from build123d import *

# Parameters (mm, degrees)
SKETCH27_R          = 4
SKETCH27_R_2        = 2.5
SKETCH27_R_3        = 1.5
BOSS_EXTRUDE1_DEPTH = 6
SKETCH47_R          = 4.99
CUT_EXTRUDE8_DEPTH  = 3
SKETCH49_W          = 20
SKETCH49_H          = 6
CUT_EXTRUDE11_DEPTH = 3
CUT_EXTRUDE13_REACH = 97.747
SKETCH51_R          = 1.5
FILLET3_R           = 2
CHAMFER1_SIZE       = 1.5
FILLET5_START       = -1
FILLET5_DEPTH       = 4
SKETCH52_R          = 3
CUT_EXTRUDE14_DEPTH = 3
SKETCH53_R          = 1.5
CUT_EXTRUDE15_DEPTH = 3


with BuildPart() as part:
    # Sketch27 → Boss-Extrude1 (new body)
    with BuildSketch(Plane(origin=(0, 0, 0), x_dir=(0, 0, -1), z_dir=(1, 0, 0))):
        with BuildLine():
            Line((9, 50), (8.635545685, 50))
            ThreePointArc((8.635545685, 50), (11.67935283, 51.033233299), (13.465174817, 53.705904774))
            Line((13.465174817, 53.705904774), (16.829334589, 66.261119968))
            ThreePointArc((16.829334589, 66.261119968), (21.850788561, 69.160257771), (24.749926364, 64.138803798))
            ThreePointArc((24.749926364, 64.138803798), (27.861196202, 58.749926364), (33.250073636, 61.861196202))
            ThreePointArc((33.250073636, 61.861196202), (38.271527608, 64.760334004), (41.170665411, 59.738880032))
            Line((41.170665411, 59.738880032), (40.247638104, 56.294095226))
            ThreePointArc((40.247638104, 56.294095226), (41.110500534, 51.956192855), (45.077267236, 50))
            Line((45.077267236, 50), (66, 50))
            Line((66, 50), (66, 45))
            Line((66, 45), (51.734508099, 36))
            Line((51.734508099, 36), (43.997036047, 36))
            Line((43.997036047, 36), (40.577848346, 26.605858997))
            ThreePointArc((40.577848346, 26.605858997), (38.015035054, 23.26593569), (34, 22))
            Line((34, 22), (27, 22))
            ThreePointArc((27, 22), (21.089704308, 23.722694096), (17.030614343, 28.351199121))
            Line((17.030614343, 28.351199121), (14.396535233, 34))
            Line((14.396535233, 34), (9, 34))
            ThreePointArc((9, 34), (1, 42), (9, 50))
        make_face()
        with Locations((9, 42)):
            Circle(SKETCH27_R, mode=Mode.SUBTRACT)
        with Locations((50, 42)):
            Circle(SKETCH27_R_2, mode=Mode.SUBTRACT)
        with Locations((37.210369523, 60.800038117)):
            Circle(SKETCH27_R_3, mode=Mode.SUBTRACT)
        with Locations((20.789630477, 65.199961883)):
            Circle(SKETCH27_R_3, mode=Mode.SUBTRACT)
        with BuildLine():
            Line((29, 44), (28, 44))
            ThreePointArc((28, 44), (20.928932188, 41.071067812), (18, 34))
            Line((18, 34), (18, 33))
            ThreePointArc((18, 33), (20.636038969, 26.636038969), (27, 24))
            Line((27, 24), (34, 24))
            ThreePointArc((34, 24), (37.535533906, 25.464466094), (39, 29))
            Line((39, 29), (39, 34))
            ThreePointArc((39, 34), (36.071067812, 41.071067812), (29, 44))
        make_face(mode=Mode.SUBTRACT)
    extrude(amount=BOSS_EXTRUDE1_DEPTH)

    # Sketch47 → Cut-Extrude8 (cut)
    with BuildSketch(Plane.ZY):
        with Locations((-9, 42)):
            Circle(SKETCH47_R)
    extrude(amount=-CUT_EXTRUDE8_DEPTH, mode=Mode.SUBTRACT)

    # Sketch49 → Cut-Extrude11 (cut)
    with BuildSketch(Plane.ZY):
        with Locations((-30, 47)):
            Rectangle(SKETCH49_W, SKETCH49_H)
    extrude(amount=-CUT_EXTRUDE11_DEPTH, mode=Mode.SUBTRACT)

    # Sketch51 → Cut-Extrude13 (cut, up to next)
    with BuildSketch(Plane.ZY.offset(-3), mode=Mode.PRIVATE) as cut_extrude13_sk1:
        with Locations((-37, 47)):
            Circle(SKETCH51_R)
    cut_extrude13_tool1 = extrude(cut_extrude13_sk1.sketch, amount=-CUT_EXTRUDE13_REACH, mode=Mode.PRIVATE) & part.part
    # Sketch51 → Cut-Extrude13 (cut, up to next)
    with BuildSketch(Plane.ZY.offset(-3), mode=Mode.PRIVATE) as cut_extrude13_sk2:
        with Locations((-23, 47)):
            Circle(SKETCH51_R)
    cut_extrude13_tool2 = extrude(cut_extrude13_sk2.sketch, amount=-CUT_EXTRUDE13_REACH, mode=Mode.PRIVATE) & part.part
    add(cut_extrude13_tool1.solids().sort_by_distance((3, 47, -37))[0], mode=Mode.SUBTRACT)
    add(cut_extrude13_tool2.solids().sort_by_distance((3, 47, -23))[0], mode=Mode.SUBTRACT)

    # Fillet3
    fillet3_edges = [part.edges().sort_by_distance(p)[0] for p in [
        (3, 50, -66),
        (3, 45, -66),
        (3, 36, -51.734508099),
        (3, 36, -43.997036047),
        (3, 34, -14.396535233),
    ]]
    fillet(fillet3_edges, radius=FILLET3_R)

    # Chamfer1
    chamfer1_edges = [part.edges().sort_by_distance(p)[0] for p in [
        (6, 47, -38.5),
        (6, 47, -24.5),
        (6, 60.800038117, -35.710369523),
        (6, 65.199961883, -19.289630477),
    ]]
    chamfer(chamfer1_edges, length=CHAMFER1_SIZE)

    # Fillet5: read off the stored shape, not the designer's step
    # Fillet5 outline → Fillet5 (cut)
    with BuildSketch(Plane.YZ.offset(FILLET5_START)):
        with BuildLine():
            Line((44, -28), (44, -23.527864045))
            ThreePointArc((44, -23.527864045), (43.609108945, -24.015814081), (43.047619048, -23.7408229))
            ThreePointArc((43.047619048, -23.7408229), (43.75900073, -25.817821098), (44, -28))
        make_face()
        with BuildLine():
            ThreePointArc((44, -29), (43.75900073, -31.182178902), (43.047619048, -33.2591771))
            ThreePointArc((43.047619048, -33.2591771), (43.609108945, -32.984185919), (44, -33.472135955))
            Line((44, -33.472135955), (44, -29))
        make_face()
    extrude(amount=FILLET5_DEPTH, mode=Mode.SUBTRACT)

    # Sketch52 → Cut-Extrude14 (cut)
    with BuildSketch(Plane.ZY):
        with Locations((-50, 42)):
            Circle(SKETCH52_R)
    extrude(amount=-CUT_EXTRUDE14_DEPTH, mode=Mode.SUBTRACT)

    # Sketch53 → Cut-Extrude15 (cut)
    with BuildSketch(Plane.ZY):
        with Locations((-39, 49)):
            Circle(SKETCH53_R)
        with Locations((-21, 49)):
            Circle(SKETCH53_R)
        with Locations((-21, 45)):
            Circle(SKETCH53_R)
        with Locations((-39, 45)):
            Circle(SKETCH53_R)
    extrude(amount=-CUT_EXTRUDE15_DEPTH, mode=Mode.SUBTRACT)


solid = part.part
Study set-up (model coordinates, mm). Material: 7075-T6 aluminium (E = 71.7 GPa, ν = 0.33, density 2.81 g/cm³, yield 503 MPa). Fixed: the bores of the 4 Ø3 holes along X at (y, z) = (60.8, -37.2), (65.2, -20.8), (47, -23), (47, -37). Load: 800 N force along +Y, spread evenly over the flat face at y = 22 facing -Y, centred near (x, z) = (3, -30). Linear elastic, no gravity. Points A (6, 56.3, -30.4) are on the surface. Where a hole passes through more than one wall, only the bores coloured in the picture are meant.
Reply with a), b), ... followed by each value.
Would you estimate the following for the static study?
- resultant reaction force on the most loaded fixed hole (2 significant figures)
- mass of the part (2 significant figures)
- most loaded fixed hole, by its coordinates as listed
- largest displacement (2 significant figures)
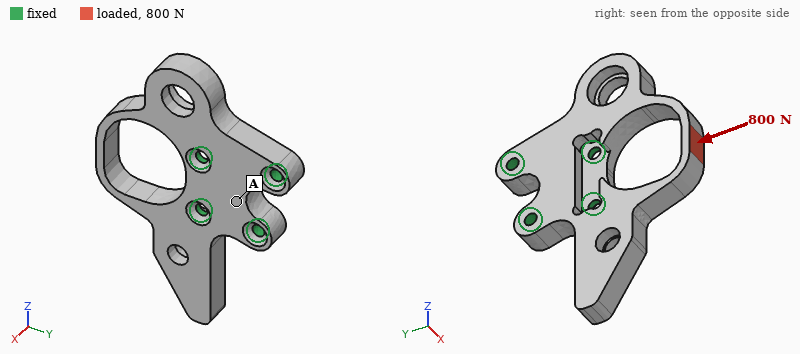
a) 610 N
b) 17 g
c) (47, -37)
d) 0.13 mm
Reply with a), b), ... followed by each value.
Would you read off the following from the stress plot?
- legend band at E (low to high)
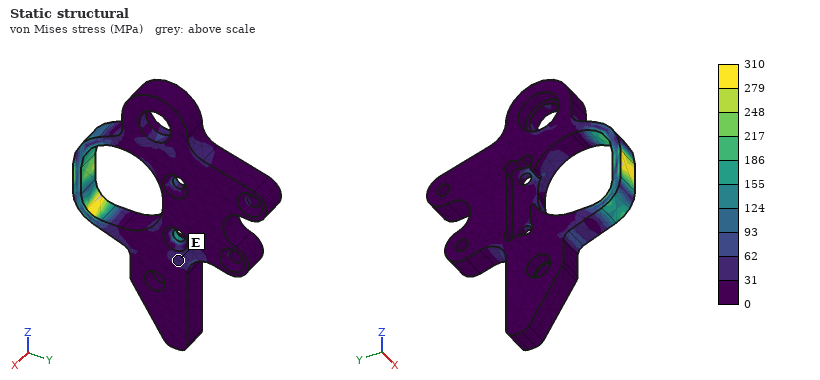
a) 31 to 62 MPa
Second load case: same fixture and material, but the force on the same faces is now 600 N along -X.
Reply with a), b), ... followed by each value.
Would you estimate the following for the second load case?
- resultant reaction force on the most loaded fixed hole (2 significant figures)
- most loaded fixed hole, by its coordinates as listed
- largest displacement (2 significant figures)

a) 780 N
b) (47, -37)
c) 0.42 mm
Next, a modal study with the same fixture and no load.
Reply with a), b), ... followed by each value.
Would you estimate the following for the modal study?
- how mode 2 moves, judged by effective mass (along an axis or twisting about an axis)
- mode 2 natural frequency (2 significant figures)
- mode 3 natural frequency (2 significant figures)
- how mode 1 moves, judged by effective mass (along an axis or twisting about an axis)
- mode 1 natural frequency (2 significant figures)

a) along X
b) 5800 Hz
c) 7200 Hz
d) along X
e) 4100 Hz
